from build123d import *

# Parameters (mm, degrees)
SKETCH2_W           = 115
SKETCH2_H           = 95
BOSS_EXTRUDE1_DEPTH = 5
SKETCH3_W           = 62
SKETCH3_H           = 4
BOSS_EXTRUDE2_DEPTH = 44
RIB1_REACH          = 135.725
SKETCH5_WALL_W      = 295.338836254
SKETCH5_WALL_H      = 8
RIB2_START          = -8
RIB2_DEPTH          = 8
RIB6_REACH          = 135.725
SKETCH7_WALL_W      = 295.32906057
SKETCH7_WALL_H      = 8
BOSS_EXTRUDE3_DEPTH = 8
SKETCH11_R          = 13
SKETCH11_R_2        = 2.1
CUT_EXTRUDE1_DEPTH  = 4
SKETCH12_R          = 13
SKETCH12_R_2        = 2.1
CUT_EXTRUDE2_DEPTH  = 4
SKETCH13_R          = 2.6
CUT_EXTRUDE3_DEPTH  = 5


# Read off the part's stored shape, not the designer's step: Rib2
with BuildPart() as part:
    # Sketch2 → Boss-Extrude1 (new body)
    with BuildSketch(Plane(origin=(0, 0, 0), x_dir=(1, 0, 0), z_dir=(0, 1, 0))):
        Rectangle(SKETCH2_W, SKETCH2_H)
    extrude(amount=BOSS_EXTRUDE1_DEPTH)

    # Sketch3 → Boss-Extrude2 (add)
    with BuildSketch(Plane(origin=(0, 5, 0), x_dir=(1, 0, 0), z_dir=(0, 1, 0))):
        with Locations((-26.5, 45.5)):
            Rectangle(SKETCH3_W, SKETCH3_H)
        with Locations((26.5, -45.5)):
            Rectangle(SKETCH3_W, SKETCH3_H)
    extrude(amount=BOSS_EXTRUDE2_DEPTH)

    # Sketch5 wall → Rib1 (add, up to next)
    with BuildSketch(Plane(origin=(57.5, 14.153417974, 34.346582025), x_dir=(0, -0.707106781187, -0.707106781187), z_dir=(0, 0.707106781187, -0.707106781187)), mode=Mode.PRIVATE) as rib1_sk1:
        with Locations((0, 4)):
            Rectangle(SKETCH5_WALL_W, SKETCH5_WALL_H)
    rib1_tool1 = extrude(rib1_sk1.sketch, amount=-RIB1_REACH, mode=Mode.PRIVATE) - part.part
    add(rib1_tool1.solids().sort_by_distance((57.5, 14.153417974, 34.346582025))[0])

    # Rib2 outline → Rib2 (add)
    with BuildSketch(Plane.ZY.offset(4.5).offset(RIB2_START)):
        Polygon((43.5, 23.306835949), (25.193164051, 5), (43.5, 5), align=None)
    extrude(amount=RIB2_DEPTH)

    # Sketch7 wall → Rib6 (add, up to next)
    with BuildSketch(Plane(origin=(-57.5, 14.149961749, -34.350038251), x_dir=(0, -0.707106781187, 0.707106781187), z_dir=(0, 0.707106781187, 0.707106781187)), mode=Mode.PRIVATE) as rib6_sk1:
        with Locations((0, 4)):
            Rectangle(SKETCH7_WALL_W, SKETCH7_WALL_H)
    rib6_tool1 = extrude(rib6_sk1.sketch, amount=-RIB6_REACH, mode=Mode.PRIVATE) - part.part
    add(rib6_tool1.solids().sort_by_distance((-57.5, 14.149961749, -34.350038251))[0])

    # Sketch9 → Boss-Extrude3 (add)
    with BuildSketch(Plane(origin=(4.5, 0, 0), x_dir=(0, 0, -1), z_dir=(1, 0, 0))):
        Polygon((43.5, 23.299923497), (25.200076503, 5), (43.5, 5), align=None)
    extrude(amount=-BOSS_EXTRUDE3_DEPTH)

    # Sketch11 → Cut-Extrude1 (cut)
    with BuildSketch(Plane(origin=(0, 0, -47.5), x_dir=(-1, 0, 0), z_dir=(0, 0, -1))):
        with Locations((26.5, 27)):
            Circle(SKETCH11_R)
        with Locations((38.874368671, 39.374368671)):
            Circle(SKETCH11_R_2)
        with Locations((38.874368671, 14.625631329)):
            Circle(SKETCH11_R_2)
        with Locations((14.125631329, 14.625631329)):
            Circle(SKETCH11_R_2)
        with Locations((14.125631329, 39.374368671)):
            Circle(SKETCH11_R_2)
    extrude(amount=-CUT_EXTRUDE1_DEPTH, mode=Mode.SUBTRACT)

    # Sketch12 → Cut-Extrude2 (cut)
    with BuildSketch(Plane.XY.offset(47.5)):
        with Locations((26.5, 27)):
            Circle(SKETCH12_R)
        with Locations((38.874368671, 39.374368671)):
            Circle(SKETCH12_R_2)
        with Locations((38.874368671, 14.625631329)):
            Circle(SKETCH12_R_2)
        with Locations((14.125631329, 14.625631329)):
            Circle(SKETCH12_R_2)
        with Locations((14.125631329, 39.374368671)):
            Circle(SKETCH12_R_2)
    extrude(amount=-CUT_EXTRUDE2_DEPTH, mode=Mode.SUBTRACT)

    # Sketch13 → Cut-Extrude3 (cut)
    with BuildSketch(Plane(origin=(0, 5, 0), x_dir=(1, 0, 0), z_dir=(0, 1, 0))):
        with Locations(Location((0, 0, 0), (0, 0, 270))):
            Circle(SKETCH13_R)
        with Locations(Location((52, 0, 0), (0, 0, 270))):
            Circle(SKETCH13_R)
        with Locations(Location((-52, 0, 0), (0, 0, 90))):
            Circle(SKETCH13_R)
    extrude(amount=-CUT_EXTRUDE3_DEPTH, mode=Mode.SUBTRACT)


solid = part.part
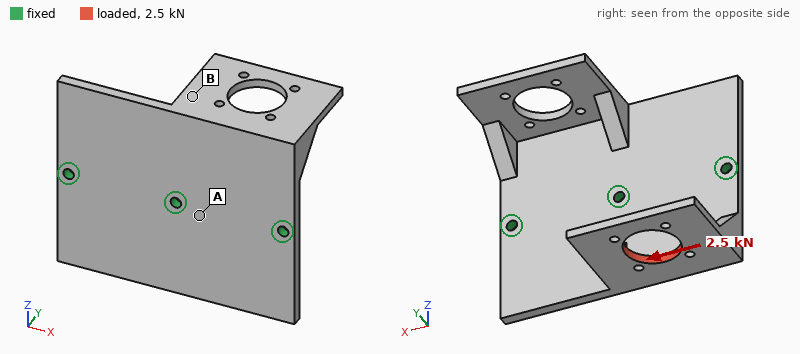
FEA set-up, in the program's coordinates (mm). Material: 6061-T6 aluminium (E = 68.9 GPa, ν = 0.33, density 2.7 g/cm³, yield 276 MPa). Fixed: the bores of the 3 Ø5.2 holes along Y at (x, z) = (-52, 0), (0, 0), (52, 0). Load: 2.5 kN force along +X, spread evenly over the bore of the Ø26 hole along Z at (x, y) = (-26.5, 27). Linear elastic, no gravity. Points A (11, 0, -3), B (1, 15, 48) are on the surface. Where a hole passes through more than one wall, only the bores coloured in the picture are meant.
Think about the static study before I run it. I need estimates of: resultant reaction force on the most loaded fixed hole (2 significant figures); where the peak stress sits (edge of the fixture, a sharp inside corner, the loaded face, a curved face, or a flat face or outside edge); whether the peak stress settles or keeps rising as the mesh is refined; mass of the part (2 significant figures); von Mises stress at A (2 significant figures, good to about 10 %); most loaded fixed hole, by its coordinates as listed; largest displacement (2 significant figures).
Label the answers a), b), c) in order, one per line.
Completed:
a) 1.7 kN
b) edge of the fixture
c) keeps rising
d) 210 g
e) 44 MPa
f) (-52, 0)
g) 0.85 mm
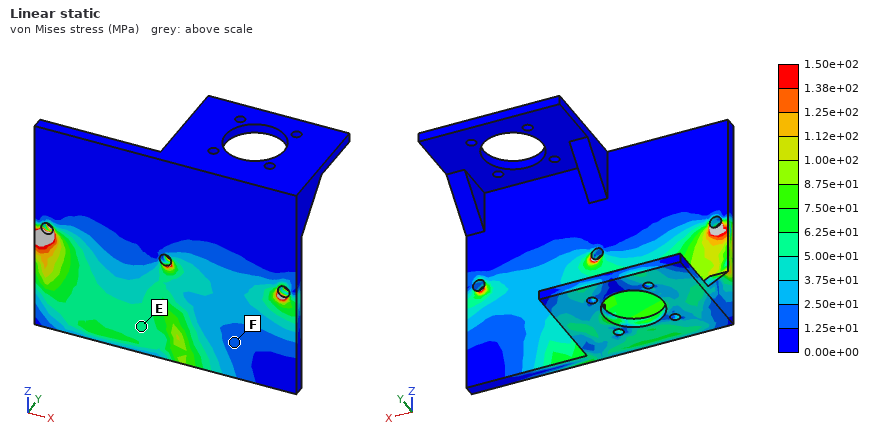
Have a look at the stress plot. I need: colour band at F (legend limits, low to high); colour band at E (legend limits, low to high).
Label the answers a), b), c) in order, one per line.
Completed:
a) 1.25e+01 to 2.50e+01 MPa
b) 5.00e+01 to 6.25e+01 MPa
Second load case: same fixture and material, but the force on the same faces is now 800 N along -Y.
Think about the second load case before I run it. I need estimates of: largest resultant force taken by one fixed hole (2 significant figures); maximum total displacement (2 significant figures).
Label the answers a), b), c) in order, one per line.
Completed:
a) 410 N
b) 0.82 mm
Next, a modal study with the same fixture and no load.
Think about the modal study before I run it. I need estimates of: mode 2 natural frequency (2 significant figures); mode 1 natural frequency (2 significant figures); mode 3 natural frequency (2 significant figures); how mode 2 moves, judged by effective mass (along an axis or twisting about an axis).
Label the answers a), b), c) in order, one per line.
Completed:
a) 960 Hz
b) 800 Hz
c) 1600 Hz
d) along Y
